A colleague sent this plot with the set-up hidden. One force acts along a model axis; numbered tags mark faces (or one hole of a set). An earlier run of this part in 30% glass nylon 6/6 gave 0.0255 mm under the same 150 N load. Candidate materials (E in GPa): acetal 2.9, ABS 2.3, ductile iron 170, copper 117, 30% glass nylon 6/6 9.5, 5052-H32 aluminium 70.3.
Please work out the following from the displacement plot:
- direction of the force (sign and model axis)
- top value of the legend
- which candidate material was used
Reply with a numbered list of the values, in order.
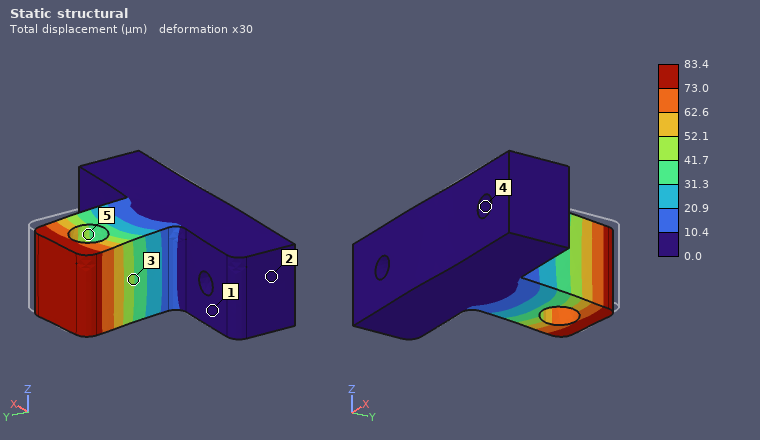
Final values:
1. -X
2. 83.4 µm
3. acetal
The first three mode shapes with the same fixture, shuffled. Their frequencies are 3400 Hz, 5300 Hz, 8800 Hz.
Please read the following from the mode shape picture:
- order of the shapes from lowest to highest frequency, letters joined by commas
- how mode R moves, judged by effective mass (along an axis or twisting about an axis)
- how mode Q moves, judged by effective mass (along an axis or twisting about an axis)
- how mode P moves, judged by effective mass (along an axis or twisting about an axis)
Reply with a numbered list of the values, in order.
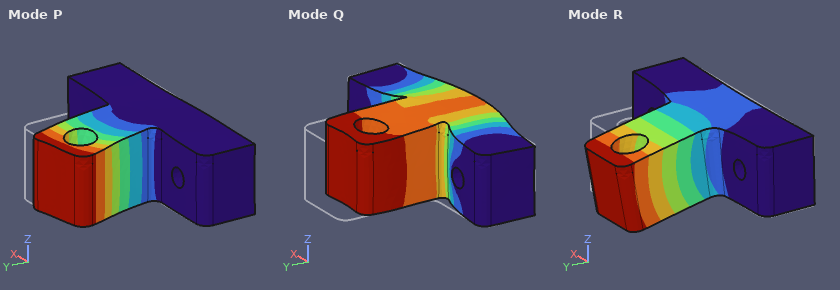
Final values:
1. R, P, Q
2. along Z
3. along Y
4. along X
